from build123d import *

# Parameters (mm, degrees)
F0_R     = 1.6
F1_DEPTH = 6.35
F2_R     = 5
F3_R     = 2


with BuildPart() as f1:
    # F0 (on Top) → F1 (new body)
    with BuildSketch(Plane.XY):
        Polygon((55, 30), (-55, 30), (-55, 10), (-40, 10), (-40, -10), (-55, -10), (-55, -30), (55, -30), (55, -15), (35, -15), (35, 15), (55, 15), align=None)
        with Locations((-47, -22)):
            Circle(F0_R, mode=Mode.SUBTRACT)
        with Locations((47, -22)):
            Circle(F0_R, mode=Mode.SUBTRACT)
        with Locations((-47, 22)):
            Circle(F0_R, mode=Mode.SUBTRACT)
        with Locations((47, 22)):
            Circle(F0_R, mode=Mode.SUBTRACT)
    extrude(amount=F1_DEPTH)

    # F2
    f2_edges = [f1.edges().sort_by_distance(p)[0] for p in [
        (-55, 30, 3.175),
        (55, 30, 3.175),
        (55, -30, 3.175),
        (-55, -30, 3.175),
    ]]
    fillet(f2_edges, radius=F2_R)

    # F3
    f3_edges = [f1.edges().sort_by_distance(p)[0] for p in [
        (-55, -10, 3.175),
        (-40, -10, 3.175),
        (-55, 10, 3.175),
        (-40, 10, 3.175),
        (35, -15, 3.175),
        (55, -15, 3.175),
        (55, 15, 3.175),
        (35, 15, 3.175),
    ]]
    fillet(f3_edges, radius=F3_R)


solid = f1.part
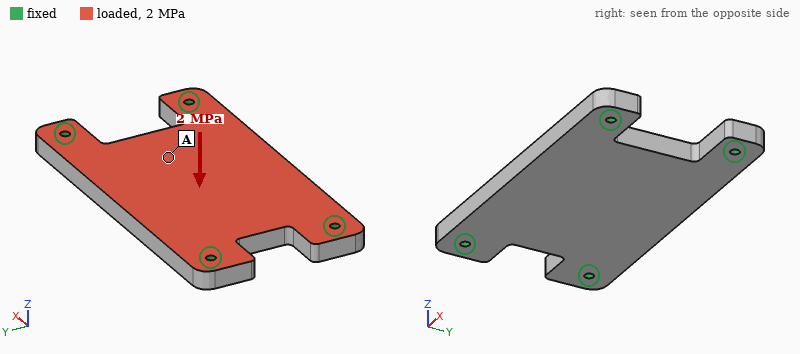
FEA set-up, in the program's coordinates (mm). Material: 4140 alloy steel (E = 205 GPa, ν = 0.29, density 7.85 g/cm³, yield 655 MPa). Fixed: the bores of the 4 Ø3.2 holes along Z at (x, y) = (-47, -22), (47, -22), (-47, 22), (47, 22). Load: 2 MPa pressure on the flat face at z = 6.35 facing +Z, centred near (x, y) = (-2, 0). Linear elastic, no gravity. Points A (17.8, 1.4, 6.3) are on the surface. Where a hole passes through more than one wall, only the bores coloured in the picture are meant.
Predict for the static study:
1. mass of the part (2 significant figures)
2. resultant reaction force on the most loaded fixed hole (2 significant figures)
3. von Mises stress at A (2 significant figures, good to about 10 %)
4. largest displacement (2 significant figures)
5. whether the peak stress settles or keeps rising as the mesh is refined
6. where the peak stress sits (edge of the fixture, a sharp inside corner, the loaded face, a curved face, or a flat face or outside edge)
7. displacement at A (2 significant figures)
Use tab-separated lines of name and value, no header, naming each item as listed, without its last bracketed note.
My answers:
mass of the part	280 g
resultant reaction force on the most loaded fixed hole	3.0 kN
von Mises stress at A	78 MPa
largest displacement	0.14 mm
whether the peak stress settles or keeps rising as the mesh is refined	keeps rising
where the peak stress sits	edge of the fixture
displacement at A	0.11 mm
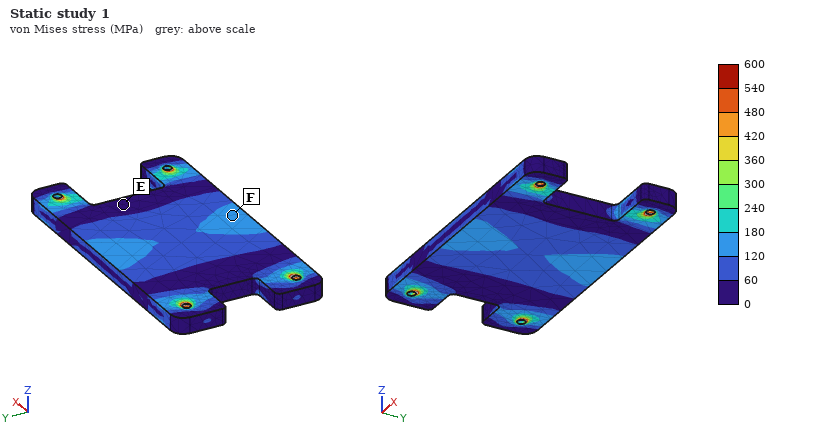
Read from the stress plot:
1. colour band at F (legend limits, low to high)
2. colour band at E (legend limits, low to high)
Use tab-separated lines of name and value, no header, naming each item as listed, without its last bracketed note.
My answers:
colour band at F	120 to 180 MPa
colour band at E	0 to 60 MPa
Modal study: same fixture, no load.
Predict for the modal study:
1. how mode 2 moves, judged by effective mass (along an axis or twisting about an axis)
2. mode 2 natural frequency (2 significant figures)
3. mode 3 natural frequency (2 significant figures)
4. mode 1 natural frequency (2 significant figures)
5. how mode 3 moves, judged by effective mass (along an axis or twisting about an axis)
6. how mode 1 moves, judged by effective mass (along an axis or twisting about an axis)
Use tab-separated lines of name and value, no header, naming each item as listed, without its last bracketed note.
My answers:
how mode 2 moves, judged by effective mass	twisting about X
mode 2 natural frequency	4800 Hz
mode 3 natural frequency	8100 Hz
mode 1 natural frequency	3000 Hz
how mode 3 moves, judged by effective mass	twisting about Y
how mode 1 moves, judged by effective mass	along Z
